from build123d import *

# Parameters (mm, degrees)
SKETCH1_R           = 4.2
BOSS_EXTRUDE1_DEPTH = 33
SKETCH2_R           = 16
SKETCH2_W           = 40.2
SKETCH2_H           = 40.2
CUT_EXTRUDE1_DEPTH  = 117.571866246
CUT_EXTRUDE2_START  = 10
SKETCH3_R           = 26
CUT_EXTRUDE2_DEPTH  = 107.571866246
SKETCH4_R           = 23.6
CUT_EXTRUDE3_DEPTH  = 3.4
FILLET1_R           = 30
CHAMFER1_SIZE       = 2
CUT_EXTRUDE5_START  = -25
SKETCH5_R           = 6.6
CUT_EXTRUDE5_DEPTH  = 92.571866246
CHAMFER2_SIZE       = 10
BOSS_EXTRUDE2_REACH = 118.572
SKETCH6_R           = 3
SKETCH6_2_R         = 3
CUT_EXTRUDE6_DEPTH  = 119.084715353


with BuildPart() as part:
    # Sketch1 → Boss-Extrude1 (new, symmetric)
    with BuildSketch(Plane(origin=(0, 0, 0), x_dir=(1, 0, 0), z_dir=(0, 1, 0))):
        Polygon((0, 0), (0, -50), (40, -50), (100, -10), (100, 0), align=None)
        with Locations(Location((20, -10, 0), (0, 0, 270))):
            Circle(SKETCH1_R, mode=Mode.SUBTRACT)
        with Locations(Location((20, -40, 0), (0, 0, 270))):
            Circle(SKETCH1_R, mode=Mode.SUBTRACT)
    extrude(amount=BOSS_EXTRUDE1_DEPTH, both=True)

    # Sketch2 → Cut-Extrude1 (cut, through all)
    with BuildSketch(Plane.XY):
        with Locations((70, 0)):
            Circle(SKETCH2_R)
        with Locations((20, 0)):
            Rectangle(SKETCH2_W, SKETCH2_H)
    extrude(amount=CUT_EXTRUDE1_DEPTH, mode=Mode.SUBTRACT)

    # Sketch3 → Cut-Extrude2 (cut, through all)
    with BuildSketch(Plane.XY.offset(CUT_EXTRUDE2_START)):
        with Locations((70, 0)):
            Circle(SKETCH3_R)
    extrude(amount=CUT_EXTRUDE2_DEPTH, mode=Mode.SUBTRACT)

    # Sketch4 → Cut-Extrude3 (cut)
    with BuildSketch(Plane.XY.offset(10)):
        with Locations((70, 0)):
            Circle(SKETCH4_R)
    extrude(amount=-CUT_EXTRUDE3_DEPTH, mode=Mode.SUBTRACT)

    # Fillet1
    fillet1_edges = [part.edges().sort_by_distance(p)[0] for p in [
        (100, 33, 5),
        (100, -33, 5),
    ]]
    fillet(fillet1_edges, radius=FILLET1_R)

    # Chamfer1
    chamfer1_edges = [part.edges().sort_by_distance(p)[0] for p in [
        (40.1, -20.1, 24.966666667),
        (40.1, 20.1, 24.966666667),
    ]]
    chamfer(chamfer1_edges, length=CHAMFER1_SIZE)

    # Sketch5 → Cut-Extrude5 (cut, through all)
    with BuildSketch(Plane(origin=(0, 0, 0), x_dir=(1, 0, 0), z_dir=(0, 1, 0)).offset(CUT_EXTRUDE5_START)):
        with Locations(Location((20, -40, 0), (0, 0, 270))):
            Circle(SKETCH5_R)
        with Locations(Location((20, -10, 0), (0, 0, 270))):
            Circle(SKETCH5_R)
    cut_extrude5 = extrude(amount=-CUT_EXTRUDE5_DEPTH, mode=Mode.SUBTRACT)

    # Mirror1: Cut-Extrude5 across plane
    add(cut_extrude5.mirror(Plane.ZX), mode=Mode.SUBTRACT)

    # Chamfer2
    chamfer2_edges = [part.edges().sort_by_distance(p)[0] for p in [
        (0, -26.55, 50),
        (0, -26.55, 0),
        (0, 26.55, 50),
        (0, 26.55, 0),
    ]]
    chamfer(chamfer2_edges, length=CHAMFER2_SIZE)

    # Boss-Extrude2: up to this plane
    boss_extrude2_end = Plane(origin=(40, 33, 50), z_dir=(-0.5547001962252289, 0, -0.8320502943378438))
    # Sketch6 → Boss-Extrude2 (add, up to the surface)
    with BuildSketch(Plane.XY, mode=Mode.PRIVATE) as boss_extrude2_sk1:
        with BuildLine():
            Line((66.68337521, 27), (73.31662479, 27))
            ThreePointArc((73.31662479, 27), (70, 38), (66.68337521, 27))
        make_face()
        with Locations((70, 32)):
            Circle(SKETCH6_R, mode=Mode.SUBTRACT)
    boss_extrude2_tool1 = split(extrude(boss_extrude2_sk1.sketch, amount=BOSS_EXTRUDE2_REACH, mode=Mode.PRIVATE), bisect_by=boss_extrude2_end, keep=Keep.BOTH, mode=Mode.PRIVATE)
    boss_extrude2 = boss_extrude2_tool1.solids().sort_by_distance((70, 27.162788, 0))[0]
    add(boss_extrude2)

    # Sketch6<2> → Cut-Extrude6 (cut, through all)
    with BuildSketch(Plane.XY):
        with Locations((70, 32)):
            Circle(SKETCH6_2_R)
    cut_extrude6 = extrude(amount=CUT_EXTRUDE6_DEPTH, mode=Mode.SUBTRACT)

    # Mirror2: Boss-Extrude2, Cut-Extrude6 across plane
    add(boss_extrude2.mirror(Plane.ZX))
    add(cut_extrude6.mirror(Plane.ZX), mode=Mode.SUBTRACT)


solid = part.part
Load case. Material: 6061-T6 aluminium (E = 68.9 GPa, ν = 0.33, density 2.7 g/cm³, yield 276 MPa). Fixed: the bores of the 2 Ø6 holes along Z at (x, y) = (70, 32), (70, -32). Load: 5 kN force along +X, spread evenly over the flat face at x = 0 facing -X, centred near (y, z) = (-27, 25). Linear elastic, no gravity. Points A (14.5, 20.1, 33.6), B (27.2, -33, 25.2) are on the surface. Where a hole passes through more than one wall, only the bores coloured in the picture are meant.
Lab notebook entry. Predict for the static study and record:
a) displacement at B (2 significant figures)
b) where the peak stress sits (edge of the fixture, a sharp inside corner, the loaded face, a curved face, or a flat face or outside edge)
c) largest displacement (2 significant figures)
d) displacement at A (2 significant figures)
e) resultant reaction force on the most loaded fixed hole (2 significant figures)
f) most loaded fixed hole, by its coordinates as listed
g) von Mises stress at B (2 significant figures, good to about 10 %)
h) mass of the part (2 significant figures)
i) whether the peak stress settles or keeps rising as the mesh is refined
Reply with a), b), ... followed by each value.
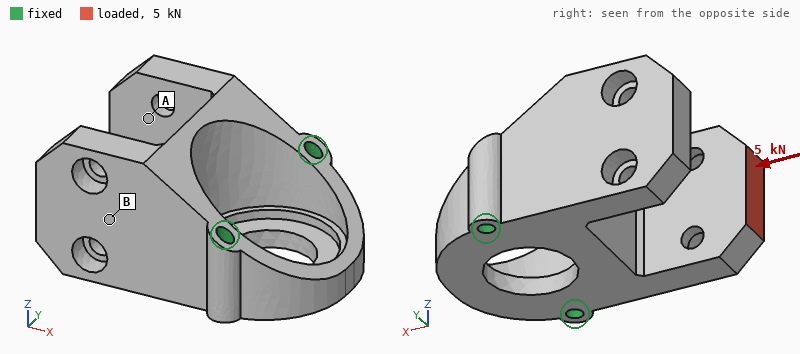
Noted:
a) 20 µm
b) edge of the fixture
c) 35 µm
d) 6.0 µm
e) 4.8 kN
f) (70, -32)
g) 17 MPa
h) 280 g
i) keeps rising
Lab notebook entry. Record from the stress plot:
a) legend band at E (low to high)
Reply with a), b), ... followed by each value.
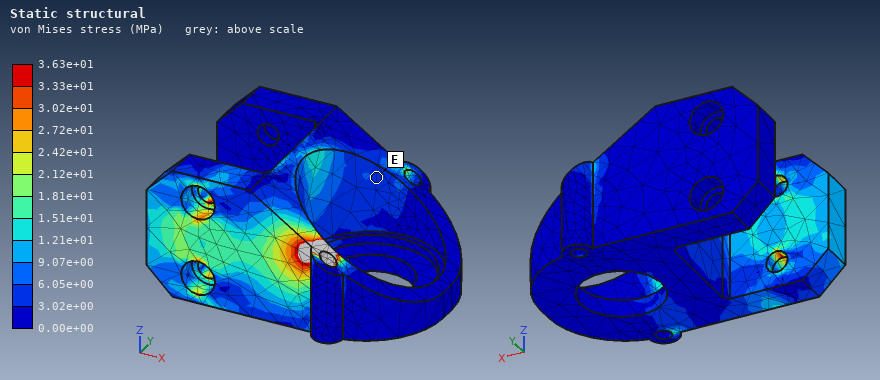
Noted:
a) 3.02e+00 to 6.05e+00 MPa
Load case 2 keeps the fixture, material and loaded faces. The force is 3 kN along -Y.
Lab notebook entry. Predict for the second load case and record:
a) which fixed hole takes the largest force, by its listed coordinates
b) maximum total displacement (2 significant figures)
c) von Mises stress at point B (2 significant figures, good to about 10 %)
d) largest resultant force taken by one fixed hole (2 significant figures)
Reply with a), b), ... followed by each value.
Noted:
a) (70, 32)
b) 0.31 mm
c) 83 MPa
d) 5.1 kN
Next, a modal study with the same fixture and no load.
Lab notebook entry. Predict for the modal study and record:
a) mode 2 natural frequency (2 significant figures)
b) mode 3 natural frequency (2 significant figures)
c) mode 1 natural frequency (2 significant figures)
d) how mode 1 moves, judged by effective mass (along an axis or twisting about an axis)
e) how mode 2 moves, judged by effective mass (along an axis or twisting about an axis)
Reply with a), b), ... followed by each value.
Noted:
a) 3900 Hz
b) 4200 Hz
c) 3100 Hz
d) along Y
e) along Z
